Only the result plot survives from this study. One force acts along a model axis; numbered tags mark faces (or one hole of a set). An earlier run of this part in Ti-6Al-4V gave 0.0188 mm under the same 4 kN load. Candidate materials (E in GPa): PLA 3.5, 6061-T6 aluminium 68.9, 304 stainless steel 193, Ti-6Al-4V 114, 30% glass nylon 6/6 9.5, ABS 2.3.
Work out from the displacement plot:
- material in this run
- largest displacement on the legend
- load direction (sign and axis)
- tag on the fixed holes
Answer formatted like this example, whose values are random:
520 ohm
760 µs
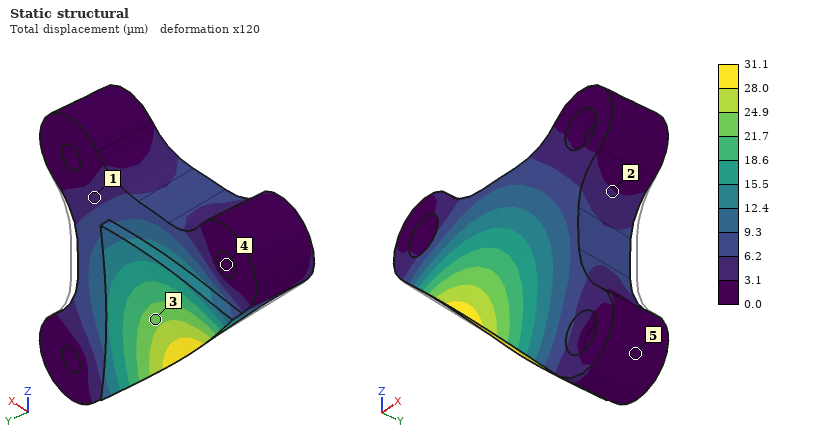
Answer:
6061-T6 aluminium
31.1 µm
-Y
4
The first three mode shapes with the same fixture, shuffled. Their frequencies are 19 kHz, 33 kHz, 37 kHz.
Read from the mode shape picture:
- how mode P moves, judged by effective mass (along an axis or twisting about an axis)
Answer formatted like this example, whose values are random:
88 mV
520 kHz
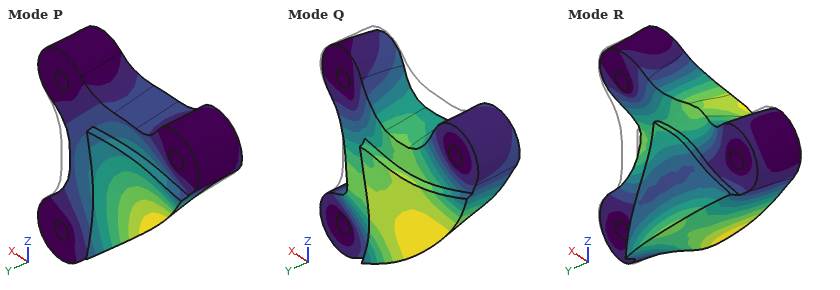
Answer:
along Y
